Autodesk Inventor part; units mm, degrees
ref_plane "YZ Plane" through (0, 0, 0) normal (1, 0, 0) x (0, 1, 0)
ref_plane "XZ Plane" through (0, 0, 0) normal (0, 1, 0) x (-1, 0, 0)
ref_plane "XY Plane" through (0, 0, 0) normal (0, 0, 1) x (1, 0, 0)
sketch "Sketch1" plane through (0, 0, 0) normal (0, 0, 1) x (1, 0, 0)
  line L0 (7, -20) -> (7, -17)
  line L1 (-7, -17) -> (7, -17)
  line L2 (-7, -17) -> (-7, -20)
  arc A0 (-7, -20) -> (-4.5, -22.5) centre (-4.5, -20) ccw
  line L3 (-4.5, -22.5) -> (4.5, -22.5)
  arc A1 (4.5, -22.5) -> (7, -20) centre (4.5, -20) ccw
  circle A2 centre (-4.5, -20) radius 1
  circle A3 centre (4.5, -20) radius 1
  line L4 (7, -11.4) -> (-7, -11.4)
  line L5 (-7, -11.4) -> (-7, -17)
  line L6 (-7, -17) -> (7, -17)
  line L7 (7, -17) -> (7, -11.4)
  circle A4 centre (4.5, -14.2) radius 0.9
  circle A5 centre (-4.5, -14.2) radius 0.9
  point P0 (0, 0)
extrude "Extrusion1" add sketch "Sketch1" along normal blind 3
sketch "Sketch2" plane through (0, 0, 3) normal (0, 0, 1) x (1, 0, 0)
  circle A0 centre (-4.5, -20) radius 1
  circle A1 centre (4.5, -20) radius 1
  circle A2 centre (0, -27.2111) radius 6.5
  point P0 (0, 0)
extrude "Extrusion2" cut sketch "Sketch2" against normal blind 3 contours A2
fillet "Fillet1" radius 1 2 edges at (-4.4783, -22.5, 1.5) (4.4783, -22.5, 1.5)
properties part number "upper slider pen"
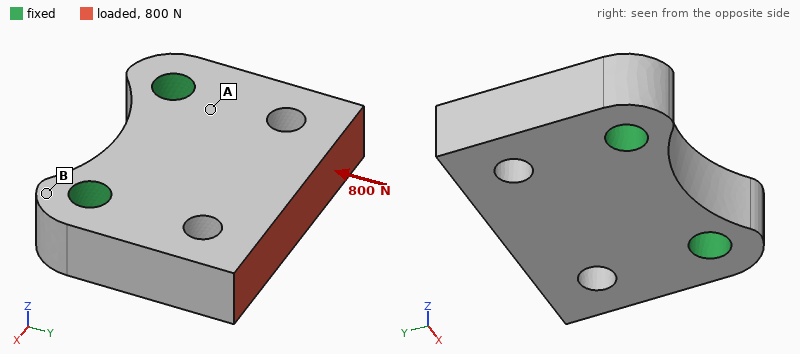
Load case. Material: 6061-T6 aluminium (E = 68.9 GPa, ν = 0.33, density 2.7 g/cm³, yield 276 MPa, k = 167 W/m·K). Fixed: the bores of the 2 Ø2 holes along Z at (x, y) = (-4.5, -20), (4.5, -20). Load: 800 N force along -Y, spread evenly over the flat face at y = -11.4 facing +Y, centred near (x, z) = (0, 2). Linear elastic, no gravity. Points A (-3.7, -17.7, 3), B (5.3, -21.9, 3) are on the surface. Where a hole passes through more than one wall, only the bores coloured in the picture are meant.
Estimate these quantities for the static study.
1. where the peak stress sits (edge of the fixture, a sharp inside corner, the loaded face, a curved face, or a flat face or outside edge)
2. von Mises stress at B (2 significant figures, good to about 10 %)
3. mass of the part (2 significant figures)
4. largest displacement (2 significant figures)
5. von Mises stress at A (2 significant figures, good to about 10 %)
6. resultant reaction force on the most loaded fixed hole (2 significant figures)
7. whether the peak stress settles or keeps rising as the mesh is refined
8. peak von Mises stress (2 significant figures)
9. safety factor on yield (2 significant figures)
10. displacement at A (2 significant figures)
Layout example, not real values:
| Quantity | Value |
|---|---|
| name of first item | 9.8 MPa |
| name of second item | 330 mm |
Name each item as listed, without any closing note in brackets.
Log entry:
| Quantity | Value |
|---|---|
| where the peak stress sits | a curved face |
| von Mises stress at B | 6.8 MPa |
| mass of the part | 1.1 g |
| largest displacement | 3.4 µm |
| von Mises stress at A | 29 MPa |
| resultant reaction force on the most loaded fixed hole | 410 N |
| whether the peak stress settles or keeps rising as the mesh is refined | settles |
| peak von Mises stress | 72 MPa |
| safety factor on yield | 3.9 |
| displacement at A | 0.73 µm |
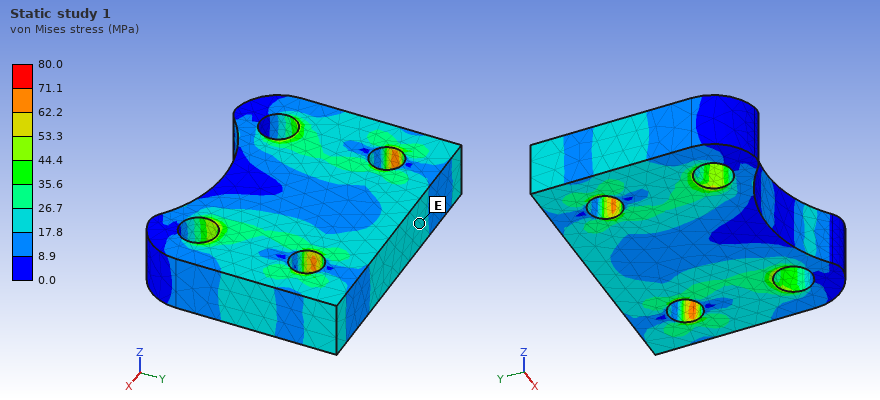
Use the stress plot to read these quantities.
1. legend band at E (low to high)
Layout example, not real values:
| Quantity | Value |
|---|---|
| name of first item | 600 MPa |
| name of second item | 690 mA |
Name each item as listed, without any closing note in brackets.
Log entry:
| Quantity | Value |
|---|---|
| legend band at E | 17.8 to 26.7 MPa |
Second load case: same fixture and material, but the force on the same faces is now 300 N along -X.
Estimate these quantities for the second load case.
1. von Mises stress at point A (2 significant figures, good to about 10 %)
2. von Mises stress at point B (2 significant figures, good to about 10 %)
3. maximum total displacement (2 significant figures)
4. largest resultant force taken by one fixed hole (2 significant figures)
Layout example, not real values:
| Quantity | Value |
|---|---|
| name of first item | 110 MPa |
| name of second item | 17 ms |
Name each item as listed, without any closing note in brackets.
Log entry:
| Quantity | Value |
|---|---|
| von Mises stress at point A | 22 MPa |
| von Mises stress at point B | 6.1 MPa |
| maximum total displacement | 5.6 µm |
| largest resultant force taken by one fixed hole | 290 N |
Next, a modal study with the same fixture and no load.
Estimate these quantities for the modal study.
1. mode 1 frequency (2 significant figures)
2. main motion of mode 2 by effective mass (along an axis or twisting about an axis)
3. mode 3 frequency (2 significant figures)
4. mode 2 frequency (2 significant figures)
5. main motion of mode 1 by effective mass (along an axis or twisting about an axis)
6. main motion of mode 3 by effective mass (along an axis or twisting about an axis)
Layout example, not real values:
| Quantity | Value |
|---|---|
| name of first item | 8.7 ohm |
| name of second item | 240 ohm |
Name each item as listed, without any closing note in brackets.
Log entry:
| Quantity | Value |
|---|---|
| mode 1 frequency | 30 kHz |
| main motion of mode 2 by effective mass | twisting about Y |
| mode 3 frequency | 72 kHz |
| mode 2 frequency | 50 kHz |
| main motion of mode 1 by effective mass | along Z |
| main motion of mode 3 by effective mass | along X |
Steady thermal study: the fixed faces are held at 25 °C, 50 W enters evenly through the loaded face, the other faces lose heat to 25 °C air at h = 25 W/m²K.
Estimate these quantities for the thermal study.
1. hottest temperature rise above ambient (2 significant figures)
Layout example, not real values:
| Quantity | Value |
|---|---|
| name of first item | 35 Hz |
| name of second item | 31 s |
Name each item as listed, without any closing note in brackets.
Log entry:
| Quantity | Value |
|---|---|
| hottest temperature rise above ambient | 69 K |
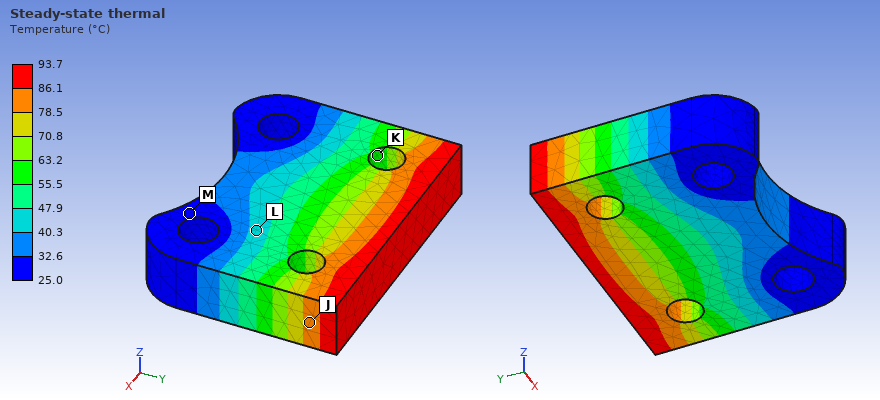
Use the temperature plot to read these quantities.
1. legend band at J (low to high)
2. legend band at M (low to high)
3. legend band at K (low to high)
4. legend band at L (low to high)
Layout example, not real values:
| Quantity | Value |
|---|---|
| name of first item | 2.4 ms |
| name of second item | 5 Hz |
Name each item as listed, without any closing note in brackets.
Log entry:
| Quantity | Value |
|---|---|
| legend band at J | 78.5 to 86.1 °C |
| legend band at M | 25.0 to 32.6 °C |
| legend band at K | 55.5 to 63.2 °C |
| legend band at L | 40.3 to 47.9 °C |
